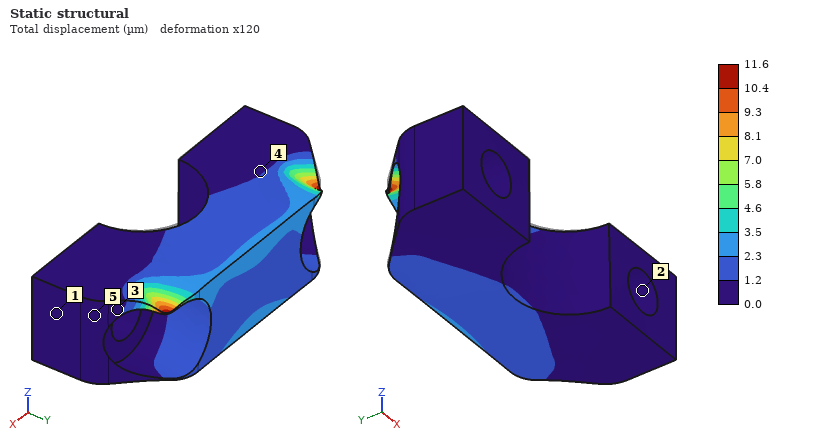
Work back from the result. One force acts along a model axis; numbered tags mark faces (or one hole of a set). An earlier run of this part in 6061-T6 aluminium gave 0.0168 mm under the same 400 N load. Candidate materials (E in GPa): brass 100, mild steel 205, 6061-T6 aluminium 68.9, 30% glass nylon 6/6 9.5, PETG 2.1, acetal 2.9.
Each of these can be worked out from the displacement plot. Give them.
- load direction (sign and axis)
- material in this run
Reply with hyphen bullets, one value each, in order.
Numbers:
- -Z
- brass
